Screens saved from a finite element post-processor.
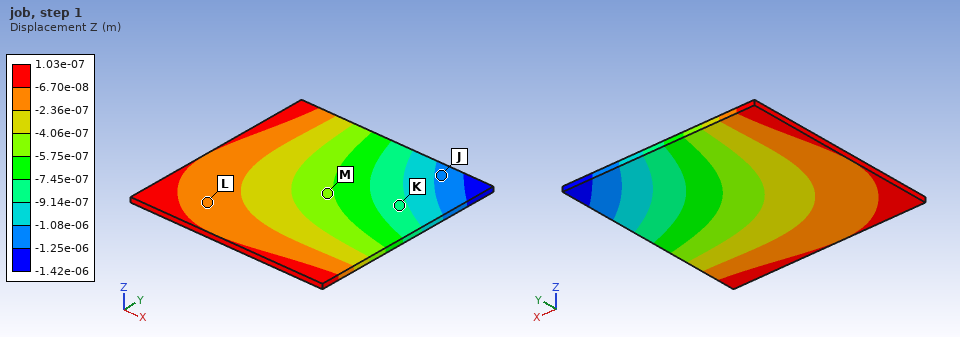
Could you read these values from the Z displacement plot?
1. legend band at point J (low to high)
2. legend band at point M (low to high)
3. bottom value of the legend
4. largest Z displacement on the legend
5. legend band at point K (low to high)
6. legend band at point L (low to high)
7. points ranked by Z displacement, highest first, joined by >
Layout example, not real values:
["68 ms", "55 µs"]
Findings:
["-1.25e-06 to -1.08e-06 m", "-5.75e-07 to -4.06e-07 m", "-1.42e-06 m", "1.03e-07 m", "-9.14e-07 to -7.45e-07 m", "-2.36e-07 to -6.70e-08 m", "L > M > K > J"]
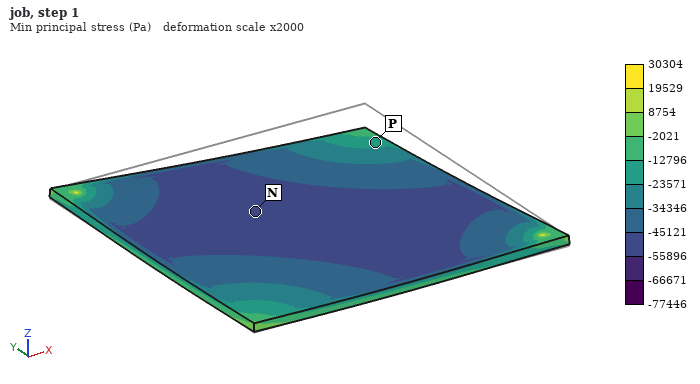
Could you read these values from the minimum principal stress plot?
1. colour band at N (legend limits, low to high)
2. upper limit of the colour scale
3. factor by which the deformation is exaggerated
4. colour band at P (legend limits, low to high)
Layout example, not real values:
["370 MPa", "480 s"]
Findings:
["-55896 to -45121 Pa", "30304 Pa", "2000", "-23571 to -12796 Pa"]
